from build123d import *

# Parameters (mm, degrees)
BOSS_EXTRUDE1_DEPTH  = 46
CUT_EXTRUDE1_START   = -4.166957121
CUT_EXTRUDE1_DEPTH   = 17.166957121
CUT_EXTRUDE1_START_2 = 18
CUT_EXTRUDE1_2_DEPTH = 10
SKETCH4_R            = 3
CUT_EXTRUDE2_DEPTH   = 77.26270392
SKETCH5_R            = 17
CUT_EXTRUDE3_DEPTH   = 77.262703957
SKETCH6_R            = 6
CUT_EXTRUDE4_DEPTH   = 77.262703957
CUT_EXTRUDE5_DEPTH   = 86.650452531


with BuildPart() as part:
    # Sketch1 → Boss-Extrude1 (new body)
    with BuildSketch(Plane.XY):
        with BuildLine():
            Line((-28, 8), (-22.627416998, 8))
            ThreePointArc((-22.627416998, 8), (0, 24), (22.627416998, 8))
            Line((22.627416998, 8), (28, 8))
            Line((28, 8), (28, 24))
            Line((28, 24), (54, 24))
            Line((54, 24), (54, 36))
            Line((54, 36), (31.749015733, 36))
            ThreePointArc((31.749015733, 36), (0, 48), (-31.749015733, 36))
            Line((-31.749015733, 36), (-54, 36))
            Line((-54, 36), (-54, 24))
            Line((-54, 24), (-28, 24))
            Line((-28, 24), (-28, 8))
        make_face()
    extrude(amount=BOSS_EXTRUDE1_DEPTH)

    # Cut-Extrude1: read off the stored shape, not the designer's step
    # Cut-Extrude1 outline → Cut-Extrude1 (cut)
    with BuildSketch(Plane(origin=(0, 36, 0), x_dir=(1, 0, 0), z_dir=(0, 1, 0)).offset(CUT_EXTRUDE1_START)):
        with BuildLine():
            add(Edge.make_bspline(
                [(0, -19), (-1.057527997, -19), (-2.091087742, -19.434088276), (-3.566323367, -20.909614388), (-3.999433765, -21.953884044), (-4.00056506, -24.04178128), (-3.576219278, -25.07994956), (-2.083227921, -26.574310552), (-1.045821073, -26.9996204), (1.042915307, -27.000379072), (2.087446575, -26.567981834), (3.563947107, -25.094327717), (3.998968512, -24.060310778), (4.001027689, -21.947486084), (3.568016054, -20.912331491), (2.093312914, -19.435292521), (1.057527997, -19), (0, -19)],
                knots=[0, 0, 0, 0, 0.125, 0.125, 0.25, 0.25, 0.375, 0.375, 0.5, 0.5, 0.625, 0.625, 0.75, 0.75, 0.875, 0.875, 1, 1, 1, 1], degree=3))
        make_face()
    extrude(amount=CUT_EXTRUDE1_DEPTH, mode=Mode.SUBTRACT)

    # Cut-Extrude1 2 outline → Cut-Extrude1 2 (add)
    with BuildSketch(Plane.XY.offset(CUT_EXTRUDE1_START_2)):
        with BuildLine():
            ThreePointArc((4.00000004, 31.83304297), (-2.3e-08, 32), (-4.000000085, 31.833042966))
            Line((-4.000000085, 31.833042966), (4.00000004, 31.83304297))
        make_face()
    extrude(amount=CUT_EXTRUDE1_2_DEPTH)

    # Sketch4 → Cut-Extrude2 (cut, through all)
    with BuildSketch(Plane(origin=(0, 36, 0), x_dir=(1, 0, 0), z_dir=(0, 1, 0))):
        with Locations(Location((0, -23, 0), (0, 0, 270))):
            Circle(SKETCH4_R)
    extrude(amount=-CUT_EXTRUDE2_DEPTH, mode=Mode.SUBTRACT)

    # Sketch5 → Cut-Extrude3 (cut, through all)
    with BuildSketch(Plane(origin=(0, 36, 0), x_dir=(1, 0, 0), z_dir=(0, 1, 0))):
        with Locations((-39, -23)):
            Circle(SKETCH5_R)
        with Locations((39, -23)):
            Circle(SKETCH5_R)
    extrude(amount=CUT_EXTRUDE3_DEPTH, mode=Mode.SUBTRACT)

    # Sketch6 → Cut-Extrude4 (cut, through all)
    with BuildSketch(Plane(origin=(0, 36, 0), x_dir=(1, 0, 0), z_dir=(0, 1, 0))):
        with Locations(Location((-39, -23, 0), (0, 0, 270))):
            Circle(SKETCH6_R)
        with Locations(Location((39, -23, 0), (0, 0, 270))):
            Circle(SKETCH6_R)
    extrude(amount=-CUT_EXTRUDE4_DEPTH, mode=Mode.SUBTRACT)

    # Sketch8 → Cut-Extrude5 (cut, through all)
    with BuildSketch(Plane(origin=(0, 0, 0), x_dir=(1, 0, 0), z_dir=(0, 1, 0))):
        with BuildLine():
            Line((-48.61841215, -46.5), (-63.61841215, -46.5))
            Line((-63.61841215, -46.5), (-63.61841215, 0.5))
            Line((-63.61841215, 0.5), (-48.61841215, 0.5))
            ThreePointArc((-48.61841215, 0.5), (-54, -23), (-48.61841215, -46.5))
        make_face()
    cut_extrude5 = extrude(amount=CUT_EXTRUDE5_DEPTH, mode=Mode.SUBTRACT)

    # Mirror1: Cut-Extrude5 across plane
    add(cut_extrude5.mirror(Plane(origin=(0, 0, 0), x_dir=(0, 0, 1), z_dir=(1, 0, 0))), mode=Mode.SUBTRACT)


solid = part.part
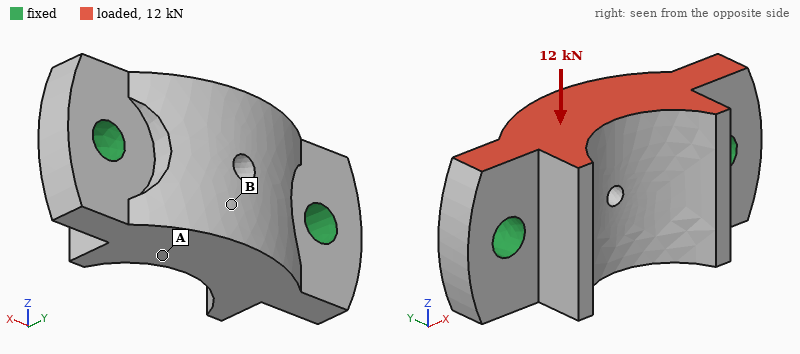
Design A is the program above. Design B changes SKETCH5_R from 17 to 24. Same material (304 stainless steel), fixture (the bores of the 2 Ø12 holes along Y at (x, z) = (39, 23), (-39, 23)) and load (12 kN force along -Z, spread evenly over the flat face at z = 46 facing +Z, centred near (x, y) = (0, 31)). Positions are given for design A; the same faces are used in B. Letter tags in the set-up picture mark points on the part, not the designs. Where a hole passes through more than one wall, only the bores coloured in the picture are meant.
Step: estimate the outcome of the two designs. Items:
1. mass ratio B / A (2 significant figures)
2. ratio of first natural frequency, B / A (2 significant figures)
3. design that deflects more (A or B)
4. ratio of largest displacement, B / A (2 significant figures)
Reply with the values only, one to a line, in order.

0.96
0.97
B
1.2
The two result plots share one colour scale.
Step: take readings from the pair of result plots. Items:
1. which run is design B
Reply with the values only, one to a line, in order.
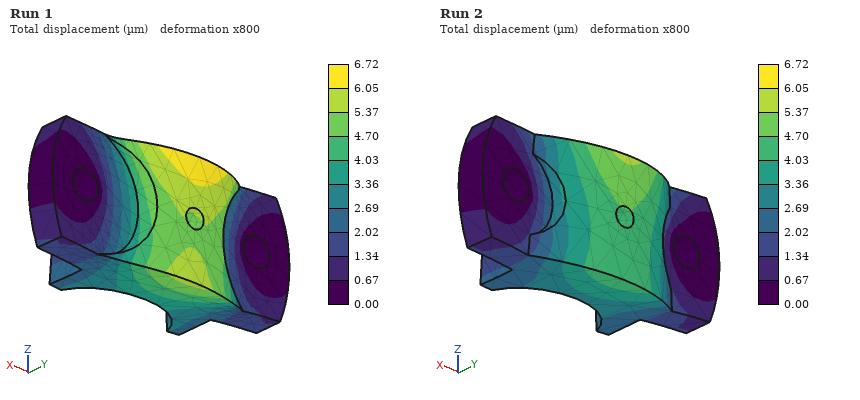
Run 1
